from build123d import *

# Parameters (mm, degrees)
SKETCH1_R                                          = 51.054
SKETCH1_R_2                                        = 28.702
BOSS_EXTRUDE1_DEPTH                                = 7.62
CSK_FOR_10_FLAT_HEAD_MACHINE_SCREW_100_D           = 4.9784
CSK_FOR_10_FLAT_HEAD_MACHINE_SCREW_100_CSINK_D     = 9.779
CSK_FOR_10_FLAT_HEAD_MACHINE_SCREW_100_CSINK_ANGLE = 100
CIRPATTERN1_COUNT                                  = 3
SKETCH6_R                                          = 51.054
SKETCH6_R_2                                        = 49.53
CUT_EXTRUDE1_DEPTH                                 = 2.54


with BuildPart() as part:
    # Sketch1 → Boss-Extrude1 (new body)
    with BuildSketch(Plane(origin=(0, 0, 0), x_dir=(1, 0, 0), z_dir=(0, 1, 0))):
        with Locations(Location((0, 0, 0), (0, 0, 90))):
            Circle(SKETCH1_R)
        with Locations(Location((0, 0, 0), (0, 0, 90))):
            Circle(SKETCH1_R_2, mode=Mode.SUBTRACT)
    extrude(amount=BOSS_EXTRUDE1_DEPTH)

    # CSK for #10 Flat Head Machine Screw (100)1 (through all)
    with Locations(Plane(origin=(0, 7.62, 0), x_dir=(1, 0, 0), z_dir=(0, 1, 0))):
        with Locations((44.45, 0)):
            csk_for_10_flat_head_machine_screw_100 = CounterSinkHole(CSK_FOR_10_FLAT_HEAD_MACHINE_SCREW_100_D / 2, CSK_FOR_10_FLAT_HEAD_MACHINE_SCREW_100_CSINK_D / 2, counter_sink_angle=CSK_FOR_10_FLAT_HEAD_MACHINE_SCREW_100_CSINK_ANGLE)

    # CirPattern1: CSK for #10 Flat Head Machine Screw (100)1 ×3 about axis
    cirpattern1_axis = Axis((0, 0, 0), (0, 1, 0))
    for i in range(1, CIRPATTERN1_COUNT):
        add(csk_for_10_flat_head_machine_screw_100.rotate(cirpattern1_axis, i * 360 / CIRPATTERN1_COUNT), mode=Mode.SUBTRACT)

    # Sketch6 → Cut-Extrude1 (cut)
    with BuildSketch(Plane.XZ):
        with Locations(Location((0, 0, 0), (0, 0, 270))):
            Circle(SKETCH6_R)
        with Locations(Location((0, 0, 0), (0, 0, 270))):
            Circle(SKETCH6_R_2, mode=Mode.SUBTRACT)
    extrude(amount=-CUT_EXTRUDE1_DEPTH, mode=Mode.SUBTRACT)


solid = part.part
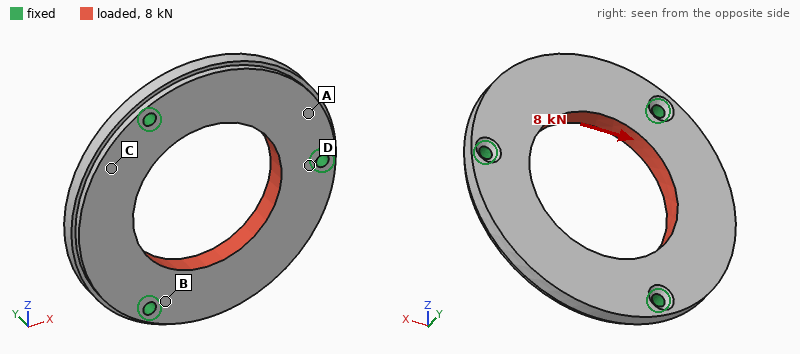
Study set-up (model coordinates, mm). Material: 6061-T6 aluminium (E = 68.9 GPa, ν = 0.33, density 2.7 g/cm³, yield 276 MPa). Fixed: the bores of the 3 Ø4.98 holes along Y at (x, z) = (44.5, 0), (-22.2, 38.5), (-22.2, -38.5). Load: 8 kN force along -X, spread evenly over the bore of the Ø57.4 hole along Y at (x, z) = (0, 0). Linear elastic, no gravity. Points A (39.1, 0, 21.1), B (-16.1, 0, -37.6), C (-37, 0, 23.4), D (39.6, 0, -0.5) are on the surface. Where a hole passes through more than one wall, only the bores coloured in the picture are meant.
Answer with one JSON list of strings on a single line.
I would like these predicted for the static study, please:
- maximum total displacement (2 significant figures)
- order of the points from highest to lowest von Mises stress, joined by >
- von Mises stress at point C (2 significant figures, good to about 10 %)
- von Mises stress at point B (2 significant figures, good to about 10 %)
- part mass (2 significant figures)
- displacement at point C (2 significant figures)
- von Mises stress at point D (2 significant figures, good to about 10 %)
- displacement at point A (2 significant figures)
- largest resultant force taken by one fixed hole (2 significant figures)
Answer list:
["16 µm", "B > D > C > A", "12 MPa", "28 MPa", "110 g", "8.9 µm", "19 MPa", "6.0 µm", "3.2 kN"]
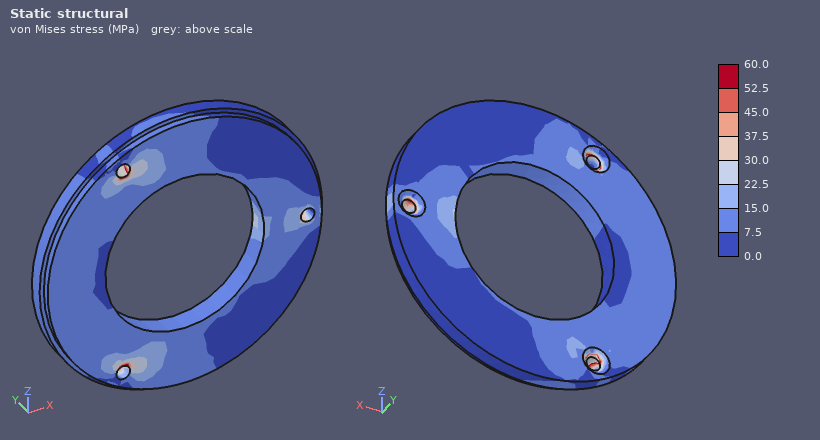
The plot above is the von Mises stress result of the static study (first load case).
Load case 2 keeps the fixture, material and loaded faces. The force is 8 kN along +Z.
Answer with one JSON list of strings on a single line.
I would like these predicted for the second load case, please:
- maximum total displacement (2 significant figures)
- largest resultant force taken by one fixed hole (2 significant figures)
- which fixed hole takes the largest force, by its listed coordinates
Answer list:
["14 µm", "3.5 kN", "(44.5, 0)"]
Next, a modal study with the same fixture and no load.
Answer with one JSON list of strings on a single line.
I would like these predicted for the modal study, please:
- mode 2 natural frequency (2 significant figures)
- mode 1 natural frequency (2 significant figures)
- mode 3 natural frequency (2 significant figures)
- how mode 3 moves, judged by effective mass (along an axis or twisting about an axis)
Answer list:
["3700 Hz", "3700 Hz", "4500 Hz", "along Y"]
